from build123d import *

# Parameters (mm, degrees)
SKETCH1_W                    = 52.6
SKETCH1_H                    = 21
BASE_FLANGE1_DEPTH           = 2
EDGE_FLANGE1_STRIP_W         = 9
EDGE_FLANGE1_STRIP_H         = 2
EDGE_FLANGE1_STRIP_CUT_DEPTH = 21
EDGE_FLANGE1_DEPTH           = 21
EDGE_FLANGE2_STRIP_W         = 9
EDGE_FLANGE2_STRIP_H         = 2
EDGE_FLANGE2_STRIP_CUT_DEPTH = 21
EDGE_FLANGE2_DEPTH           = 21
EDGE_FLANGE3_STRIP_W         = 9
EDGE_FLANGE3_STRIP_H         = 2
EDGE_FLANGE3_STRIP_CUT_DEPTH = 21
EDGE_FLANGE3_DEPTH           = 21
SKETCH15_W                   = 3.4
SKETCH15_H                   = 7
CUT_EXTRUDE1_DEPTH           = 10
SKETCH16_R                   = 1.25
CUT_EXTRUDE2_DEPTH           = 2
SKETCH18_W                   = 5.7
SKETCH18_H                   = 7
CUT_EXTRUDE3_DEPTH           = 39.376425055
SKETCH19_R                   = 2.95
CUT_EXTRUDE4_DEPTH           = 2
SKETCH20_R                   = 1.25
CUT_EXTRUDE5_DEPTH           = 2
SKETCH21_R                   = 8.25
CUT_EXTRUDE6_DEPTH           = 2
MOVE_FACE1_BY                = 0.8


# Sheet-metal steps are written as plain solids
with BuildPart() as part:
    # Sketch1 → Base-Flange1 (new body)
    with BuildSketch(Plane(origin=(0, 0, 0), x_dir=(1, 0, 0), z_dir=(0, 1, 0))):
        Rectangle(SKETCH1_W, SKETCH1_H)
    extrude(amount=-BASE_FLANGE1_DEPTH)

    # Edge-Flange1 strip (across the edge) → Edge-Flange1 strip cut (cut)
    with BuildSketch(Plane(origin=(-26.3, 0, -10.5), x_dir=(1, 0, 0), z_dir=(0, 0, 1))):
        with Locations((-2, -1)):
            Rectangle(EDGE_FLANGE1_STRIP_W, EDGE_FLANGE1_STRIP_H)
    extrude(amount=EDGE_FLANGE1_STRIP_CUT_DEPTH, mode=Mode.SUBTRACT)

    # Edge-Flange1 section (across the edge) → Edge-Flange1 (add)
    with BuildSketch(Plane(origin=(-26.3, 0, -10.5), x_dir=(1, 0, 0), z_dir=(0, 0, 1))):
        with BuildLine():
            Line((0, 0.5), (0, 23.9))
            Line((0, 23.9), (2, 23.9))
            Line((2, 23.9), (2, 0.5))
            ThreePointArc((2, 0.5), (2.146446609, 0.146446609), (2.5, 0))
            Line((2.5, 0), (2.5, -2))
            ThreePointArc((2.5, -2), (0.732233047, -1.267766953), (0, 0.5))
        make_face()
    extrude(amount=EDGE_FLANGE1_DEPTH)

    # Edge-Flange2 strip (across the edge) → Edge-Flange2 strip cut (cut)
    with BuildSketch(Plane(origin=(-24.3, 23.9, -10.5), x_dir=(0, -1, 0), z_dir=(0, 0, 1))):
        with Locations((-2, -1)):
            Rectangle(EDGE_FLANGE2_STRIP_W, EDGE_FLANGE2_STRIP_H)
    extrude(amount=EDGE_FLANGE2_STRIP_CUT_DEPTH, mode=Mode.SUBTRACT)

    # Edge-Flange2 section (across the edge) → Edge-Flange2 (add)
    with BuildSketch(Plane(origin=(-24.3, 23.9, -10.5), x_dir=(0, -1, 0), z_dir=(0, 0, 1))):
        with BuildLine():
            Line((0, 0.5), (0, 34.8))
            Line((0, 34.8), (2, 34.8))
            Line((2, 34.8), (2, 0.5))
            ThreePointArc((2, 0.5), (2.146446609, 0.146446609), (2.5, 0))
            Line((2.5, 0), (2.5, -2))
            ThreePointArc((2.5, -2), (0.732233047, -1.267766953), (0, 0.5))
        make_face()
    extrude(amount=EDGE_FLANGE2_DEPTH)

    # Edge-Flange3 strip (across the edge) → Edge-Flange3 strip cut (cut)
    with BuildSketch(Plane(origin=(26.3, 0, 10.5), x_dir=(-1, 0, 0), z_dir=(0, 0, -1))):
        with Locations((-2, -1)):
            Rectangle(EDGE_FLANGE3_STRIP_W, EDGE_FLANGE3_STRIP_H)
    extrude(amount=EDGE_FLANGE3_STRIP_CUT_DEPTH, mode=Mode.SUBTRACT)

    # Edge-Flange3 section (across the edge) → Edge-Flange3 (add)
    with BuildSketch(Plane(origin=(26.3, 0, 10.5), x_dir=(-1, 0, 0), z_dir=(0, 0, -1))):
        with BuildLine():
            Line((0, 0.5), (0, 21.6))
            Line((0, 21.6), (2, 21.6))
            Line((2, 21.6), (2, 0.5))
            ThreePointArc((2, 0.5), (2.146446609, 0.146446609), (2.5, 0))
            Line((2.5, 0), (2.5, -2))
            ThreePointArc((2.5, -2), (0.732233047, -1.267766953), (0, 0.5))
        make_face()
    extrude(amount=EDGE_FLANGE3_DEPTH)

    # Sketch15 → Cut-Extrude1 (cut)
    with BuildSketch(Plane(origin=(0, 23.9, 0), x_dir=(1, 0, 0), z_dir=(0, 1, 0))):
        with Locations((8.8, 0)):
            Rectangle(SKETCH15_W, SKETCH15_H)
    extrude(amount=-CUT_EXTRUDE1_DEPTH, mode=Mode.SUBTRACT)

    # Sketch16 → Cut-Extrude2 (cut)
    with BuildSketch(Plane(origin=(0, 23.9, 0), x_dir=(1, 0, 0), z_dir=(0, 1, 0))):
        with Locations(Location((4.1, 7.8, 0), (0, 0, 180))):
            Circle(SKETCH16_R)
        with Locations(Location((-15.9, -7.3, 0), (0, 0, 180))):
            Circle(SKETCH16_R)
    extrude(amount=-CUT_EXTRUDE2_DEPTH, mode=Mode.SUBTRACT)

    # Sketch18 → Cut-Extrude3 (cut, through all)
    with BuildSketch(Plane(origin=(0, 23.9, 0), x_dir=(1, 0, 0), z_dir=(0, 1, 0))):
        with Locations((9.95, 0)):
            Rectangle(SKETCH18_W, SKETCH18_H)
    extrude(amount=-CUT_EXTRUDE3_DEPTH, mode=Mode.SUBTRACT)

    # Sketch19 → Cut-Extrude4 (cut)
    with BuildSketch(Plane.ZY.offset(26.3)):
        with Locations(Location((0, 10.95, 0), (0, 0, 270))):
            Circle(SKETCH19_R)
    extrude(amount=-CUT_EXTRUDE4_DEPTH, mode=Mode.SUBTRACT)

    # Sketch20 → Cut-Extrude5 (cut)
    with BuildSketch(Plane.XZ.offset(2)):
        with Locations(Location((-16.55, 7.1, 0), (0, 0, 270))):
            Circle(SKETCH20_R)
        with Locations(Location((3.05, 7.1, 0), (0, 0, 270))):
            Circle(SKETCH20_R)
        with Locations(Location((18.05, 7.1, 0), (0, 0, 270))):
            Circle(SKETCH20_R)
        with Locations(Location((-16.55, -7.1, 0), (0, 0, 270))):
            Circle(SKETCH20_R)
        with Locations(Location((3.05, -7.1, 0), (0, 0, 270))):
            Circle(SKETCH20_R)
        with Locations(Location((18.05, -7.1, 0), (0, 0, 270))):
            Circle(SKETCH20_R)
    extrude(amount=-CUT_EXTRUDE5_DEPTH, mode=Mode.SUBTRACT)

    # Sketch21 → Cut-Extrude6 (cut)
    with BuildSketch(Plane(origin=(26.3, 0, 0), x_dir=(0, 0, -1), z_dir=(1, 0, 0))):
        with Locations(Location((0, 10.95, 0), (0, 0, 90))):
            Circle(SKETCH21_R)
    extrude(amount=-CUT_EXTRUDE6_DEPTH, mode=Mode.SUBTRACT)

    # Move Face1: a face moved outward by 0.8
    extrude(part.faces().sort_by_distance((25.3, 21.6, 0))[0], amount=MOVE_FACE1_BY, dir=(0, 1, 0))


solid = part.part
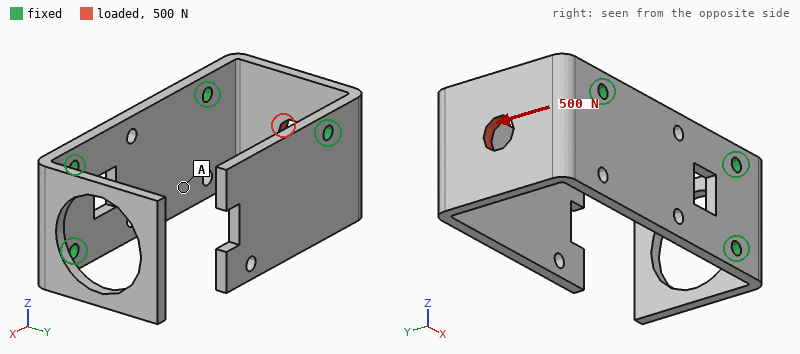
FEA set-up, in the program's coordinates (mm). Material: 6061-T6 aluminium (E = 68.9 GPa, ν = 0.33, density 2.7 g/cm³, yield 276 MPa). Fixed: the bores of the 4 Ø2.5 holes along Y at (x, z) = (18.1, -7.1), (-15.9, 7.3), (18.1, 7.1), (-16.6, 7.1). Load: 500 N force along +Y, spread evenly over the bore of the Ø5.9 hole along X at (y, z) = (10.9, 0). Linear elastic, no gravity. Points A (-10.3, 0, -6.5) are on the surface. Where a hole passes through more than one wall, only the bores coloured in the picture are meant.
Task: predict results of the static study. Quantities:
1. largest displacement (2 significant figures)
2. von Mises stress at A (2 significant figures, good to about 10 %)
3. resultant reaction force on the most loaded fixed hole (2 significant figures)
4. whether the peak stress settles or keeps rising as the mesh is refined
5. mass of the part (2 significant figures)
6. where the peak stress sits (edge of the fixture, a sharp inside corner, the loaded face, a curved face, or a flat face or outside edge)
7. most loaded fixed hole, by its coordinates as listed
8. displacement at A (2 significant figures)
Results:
57 µm
15 MPa
320 N
keeps rising
13 g
edge of the fixture
(-16.6, 7.1)
13 µm
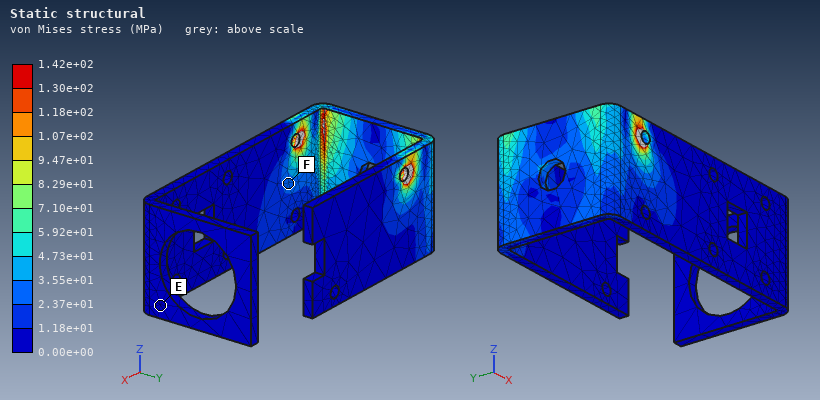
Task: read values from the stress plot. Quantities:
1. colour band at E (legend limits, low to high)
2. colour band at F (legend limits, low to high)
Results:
0.00e+00 to 1.18e+01 MPa
2.37e+01 to 3.55e+01 MPa
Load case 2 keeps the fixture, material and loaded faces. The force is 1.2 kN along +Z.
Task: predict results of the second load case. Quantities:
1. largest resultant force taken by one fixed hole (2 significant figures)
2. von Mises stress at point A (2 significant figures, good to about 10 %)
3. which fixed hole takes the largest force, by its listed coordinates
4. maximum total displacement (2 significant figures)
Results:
760 N
20 MPa
(-16.6, 7.1)
0.16 mm
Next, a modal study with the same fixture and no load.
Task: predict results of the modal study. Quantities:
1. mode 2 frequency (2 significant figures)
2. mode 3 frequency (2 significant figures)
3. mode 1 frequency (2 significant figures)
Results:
2100 Hz
4700 Hz
2000 Hz
